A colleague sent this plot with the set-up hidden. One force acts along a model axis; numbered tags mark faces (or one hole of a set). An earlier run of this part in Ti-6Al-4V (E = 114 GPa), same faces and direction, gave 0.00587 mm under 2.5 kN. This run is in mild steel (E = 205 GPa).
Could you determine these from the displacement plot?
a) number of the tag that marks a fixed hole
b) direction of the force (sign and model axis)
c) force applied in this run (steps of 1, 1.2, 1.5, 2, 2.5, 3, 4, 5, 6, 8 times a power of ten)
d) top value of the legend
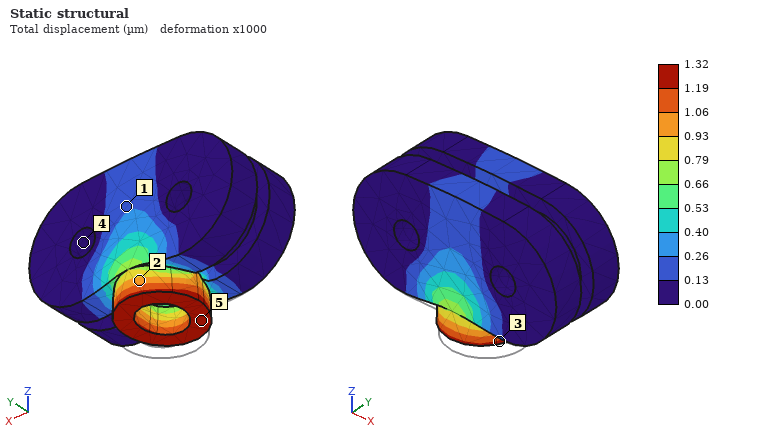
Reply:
4
+Z
1 kN
1.32 µm
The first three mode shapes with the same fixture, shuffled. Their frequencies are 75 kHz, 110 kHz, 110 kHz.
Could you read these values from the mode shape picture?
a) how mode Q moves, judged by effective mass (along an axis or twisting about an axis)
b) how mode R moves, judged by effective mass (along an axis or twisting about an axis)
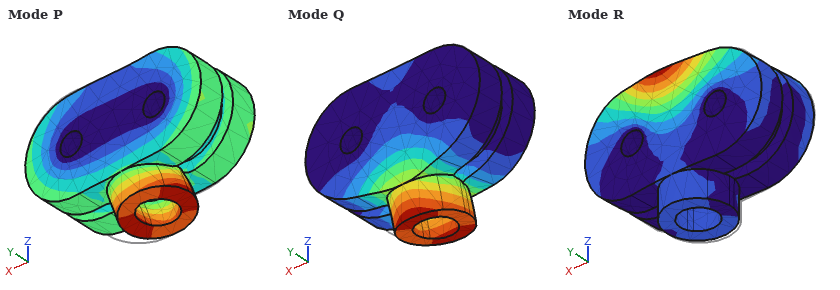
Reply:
along Y
along Y
